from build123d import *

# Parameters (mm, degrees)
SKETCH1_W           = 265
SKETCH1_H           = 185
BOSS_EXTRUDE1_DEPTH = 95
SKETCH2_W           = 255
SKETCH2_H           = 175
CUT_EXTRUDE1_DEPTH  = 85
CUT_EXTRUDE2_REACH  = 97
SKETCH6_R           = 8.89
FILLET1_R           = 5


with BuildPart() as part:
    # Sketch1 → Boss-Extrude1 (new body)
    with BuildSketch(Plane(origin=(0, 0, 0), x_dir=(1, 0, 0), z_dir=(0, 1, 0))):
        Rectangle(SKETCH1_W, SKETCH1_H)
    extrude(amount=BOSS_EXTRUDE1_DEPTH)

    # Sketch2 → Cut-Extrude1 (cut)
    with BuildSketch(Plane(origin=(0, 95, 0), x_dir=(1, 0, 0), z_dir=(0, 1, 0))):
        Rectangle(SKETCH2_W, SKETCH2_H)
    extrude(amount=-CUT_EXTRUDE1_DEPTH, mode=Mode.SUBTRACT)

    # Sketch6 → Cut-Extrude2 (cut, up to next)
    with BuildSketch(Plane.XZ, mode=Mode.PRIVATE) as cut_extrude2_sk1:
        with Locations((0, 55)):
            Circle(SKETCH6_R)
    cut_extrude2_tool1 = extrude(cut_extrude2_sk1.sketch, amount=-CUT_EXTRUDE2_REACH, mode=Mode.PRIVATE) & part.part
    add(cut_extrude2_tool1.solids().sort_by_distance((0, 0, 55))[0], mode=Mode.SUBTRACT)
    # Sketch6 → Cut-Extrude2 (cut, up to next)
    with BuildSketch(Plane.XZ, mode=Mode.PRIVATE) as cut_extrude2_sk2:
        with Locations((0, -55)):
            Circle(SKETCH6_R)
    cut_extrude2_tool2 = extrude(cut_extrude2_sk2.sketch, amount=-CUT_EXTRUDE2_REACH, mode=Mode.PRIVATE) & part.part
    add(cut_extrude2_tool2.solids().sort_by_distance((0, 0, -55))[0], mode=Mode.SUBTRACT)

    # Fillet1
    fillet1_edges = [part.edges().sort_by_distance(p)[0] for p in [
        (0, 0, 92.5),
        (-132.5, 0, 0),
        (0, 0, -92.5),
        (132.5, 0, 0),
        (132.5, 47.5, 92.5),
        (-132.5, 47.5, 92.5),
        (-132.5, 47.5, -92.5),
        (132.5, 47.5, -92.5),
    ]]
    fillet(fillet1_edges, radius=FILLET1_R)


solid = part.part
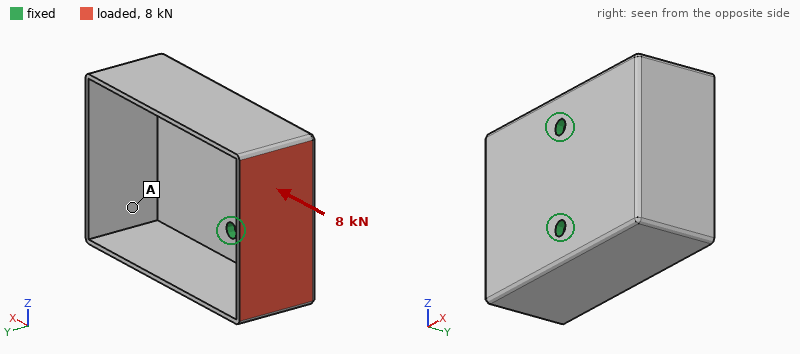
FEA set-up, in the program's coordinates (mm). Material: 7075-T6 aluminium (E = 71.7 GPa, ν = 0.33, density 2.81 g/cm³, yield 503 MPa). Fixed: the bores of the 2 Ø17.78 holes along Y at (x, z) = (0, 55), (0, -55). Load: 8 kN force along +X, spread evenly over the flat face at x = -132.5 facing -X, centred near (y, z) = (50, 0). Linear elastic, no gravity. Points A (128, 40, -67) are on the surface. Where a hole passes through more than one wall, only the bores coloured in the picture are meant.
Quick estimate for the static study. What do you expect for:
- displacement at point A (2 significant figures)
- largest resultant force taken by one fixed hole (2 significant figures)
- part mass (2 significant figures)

0.52 mm
4.1 kN
2.4 kg
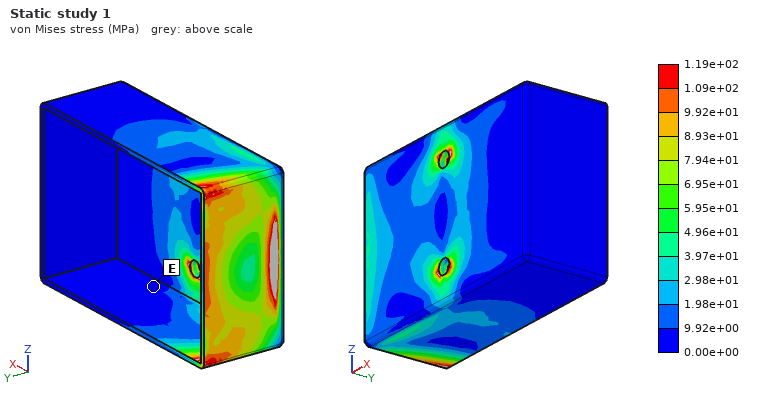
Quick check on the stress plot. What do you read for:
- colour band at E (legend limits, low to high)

0.00e+00 to 9.92e+00 MPa
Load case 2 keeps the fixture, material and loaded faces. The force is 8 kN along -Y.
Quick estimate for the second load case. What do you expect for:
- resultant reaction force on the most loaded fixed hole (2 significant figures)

4.1 kN
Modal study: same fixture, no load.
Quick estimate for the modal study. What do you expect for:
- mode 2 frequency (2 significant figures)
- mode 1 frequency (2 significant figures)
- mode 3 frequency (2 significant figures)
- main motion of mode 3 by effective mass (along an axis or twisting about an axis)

440 Hz
340 Hz
680 Hz
along Z
